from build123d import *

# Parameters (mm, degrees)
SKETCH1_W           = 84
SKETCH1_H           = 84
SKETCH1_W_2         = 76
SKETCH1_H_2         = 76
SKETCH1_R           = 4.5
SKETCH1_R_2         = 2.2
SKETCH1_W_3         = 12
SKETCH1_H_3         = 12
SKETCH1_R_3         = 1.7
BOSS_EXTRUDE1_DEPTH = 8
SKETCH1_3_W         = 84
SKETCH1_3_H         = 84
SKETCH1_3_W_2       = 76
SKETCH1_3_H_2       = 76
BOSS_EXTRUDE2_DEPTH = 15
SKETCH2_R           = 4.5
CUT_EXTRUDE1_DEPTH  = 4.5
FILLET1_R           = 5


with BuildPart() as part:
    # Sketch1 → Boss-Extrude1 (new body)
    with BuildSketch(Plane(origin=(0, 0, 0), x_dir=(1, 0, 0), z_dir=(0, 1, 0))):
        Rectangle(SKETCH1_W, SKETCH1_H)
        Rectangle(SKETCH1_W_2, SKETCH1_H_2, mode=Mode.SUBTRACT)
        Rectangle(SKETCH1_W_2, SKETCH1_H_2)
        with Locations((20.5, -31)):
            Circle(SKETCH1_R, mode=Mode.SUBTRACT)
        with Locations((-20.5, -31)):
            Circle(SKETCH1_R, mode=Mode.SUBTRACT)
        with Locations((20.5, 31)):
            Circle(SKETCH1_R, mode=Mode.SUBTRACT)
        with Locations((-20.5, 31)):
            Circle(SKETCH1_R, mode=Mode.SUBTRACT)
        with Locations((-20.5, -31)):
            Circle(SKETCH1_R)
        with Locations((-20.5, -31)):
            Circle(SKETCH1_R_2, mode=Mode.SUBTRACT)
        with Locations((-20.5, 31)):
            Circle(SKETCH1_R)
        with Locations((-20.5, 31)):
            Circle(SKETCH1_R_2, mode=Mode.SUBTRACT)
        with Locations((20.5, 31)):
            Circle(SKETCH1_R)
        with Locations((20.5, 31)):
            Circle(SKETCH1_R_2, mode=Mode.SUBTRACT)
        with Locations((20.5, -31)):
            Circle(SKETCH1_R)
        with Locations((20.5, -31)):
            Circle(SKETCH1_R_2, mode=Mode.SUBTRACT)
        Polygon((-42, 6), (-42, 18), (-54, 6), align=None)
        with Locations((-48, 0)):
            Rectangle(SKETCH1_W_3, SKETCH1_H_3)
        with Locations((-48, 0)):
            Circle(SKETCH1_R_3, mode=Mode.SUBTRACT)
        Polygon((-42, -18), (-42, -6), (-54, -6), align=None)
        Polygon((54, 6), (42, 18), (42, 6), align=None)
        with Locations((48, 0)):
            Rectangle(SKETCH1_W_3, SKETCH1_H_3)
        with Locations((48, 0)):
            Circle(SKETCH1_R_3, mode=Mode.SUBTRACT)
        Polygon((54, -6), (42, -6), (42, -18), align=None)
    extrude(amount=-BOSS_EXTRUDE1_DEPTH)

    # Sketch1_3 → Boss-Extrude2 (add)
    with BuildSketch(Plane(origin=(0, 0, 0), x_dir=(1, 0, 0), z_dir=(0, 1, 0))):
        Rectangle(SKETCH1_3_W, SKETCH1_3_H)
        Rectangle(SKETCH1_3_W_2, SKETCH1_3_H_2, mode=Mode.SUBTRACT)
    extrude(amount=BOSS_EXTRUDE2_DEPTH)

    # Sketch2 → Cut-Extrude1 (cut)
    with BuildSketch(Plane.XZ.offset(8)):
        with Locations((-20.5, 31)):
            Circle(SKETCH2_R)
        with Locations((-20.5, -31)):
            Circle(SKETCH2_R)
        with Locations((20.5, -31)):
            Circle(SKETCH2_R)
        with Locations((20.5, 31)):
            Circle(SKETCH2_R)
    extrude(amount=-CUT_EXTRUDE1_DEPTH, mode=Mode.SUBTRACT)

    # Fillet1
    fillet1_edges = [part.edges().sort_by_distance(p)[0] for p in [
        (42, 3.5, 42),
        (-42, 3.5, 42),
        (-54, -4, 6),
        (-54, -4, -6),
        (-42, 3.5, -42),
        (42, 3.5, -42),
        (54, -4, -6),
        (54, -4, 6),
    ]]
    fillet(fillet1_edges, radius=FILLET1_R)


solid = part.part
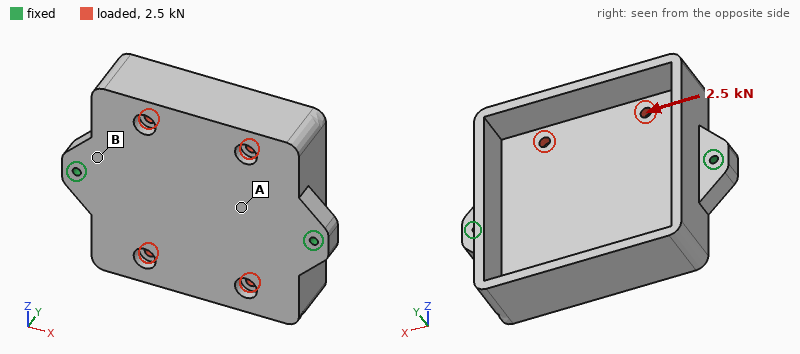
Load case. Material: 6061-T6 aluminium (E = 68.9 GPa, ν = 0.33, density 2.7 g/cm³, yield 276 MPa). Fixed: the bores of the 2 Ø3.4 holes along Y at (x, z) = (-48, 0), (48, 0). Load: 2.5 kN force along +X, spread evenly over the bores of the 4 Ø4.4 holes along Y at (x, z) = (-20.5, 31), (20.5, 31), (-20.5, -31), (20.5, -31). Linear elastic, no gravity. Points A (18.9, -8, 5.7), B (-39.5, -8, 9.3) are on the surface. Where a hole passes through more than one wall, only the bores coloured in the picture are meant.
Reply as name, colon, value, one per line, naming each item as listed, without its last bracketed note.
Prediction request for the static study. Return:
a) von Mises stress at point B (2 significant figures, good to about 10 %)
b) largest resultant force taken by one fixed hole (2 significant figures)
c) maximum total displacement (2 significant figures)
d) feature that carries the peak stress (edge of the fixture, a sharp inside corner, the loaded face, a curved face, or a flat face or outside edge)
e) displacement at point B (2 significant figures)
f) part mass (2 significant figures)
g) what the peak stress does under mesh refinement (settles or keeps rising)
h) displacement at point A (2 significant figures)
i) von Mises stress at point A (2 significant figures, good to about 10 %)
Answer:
von Mises stress at point B: 5.0 MPa
largest resultant force taken by one fixed hole: 1.3 kN
maximum total displacement: 5.4 µm
feature that carries the peak stress: edge of the fixture
displacement at point B: 1.9 µm
part mass: 210 g
what the peak stress does under mesh refinement: keeps rising
displacement at point A: 2.5 µm
von Mises stress at point A: 2.3 MPa
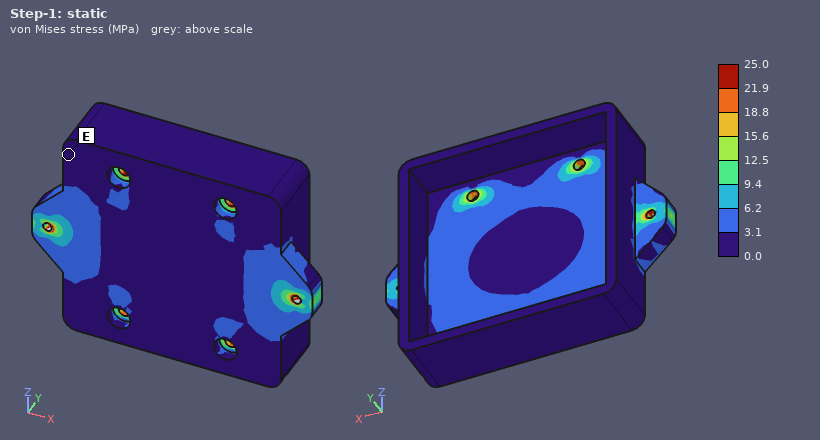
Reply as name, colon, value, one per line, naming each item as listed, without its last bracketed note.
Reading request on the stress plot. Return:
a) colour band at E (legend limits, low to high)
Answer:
colour band at E: 0.0 to 3.1 MPa
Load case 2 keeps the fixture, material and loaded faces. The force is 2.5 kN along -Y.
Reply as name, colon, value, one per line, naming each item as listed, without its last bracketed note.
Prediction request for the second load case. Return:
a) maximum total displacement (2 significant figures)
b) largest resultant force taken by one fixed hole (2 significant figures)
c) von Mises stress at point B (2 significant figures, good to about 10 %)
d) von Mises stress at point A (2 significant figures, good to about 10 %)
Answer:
maximum total displacement: 53 µm
largest resultant force taken by one fixed hole: 1.3 kN
von Mises stress at point B: 14 MPa
von Mises stress at point A: 12 MPa
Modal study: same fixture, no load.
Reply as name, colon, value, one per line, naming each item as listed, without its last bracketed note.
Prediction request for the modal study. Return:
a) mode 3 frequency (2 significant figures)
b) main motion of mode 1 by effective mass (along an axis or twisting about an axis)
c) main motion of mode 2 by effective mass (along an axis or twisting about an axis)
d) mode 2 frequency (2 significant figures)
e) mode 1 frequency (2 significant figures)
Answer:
mode 3 frequency: 3700 Hz
main motion of mode 1 by effective mass: twisting about X
main motion of mode 2 by effective mass: along Y
mode 2 frequency: 3100 Hz
mode 1 frequency: 1600 Hz
